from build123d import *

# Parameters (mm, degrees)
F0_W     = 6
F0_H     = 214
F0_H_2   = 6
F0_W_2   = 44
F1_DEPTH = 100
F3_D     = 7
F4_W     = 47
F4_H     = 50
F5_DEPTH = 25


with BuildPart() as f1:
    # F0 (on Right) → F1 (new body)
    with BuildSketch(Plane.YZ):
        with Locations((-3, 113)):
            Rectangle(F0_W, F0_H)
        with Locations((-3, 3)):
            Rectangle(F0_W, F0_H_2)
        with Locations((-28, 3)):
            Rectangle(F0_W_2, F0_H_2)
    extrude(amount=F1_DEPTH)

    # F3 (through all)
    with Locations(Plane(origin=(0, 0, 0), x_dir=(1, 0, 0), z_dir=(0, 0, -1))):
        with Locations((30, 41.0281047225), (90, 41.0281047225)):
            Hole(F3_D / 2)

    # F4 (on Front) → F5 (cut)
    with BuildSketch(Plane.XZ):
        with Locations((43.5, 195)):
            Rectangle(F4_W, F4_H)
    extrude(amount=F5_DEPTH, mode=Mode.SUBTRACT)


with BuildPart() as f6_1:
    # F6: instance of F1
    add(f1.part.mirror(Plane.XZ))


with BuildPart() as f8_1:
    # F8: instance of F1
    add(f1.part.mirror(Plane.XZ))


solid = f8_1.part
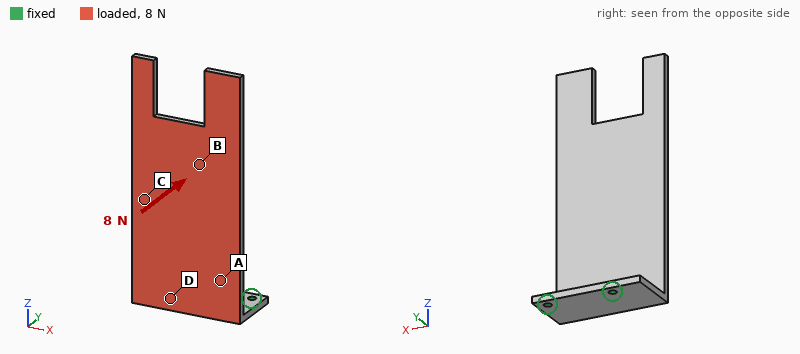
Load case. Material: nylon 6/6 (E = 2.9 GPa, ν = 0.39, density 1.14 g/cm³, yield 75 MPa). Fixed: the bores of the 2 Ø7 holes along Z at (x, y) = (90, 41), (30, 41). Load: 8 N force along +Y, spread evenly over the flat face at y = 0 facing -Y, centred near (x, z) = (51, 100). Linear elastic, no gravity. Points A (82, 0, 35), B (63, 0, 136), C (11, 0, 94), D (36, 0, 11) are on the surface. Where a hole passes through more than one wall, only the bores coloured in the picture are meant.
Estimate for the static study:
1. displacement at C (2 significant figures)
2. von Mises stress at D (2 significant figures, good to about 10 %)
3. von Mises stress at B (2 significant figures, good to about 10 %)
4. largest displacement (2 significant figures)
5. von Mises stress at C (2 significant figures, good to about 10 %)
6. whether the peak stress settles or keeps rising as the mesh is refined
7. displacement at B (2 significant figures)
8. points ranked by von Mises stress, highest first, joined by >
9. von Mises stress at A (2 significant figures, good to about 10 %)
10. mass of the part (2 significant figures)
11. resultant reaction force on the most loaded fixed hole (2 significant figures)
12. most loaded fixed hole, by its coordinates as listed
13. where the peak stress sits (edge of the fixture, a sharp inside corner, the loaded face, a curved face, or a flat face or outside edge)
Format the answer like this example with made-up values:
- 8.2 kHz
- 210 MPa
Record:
- 0.91 mm
- 1.1 MPa
- 0.16 MPa
- 2.7 mm
- 0.38 MPa
- keeps rising
- 1.5 mm
- D > A > C > B
- 0.85 MPa
- 160 g
- 6.2 N
- (30, 41)
- edge of the fixture
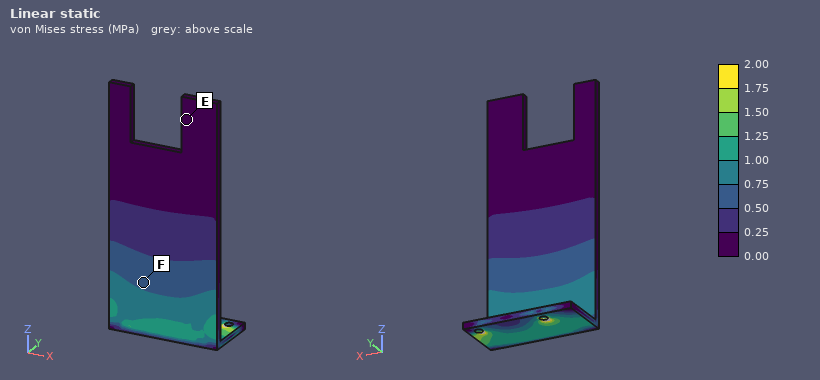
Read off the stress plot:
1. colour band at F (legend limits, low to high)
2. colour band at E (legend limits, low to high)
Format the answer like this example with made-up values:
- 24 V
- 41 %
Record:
- 0.50 to 0.75 MPa
- 0.00 to 0.25 MPa
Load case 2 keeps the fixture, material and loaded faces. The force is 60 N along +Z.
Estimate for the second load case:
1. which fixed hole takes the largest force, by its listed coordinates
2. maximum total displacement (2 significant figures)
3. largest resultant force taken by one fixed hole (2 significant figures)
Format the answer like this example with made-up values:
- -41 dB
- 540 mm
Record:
- (30, 41)
- 2.8 mm
- 38 N
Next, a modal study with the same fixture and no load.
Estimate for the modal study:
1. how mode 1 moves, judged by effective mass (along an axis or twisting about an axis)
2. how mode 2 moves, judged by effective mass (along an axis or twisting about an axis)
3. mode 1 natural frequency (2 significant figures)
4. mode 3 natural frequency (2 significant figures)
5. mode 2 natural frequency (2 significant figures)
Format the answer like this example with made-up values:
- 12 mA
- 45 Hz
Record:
- along Y
- along X
- 31 Hz
- 140 Hz
- 86 Hz
